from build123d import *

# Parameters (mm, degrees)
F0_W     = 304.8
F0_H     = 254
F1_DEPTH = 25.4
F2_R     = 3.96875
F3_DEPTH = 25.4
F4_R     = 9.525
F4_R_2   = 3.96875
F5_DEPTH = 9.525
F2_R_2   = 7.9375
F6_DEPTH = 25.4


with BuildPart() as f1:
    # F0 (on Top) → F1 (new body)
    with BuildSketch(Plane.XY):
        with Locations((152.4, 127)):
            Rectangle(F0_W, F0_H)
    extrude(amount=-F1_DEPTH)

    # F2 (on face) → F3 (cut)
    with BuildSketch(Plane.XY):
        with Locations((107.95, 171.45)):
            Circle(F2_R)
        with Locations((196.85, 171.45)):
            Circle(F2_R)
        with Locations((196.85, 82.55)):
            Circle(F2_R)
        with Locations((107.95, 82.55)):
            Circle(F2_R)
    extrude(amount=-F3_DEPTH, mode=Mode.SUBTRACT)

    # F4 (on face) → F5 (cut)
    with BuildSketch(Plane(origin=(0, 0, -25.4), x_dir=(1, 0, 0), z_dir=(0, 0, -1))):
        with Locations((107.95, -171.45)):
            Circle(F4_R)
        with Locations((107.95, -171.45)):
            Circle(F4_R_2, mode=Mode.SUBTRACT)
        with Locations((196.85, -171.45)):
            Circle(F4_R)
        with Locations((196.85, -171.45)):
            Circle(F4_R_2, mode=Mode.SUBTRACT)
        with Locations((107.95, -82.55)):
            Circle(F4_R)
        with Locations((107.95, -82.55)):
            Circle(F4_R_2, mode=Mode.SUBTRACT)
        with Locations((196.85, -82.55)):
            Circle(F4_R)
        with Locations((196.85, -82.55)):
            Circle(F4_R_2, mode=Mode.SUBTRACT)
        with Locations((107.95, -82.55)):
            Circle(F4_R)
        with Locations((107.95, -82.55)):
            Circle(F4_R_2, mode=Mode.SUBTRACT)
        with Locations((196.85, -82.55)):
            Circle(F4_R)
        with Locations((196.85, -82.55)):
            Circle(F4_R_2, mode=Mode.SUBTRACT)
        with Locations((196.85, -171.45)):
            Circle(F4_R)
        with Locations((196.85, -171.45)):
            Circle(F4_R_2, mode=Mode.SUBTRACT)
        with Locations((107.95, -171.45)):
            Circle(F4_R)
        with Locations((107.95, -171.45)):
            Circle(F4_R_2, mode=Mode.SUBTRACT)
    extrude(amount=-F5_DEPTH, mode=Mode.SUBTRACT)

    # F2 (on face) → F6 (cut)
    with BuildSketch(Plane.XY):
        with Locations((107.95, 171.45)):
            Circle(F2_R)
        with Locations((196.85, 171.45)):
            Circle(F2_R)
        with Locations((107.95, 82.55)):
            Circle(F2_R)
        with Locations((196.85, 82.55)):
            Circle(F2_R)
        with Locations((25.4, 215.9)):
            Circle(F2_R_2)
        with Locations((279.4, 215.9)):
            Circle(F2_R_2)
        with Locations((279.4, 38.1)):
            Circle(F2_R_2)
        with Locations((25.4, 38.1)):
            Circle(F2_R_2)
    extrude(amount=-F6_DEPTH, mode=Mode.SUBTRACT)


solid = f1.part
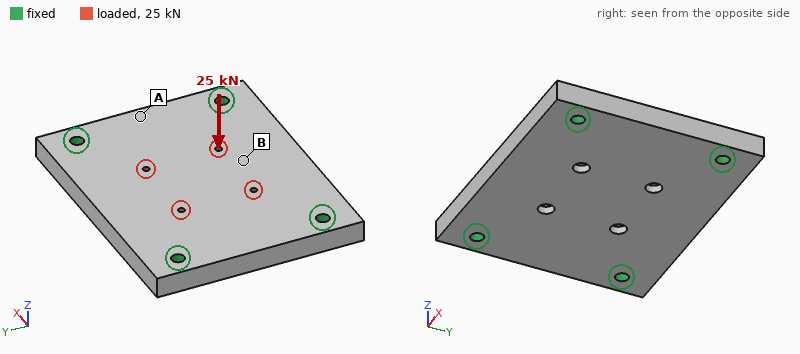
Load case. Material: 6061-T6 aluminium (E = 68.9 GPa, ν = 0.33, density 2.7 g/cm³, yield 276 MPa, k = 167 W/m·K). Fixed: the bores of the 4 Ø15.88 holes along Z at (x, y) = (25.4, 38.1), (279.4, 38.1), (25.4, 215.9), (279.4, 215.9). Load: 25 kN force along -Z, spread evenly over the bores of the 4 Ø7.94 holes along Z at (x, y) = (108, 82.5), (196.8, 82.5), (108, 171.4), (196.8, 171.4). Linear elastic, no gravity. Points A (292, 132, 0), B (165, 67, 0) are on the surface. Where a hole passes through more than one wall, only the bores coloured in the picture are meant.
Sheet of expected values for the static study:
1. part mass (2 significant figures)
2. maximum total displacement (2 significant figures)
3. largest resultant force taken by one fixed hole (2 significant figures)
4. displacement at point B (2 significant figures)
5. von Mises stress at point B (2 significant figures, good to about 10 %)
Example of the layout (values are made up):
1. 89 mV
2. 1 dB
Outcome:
1. 5.2 kg
2. 0.13 mm
3. 6.3 kN
4. 0.11 mm
5. 15 MPa
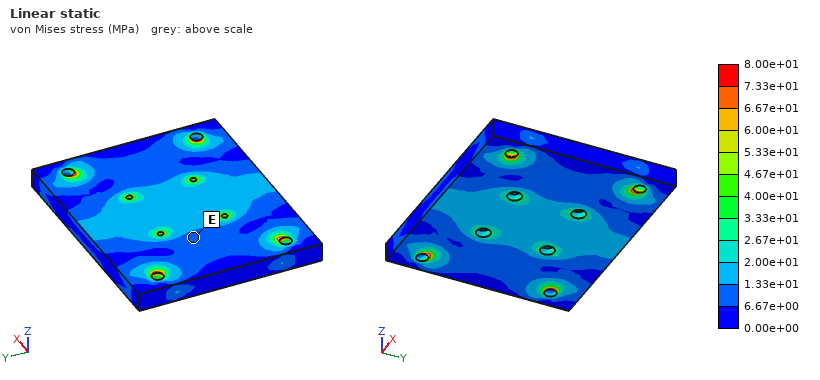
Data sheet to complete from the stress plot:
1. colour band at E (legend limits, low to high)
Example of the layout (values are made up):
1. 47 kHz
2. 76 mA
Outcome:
1. 6.67e+00 to 1.33e+01 MPa
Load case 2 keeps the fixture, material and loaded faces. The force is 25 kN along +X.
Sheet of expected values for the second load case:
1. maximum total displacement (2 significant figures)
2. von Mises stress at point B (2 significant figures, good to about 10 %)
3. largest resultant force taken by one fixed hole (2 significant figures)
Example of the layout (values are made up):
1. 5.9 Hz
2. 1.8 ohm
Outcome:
1. 8.7 µm
2. 2.9 MPa
3. 6.6 kN
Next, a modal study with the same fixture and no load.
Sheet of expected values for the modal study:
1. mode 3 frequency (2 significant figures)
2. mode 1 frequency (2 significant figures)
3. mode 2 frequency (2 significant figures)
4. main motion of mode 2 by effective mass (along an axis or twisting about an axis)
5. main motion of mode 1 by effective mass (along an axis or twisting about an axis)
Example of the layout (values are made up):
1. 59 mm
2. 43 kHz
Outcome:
1. 3000 Hz
2. 1600 Hz
3. 2200 Hz
4. twisting about X
5. along Z
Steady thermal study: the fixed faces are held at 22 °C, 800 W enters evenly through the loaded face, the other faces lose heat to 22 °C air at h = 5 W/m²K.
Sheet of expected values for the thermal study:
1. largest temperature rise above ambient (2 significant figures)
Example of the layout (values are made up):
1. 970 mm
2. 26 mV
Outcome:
1. 63 K
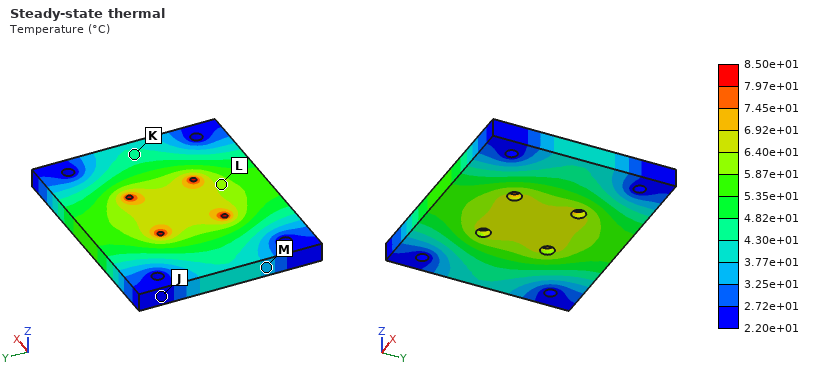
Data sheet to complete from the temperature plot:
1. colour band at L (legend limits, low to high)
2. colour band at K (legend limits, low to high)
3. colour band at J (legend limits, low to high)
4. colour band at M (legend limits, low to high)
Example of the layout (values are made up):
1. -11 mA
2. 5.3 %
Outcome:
1. 5.87e+01 to 6.40e+01 °C
2. 4.30e+01 to 4.82e+01 °C
3. 2.20e+01 to 2.72e+01 °C
4. 3.25e+01 to 3.77e+01 °C
